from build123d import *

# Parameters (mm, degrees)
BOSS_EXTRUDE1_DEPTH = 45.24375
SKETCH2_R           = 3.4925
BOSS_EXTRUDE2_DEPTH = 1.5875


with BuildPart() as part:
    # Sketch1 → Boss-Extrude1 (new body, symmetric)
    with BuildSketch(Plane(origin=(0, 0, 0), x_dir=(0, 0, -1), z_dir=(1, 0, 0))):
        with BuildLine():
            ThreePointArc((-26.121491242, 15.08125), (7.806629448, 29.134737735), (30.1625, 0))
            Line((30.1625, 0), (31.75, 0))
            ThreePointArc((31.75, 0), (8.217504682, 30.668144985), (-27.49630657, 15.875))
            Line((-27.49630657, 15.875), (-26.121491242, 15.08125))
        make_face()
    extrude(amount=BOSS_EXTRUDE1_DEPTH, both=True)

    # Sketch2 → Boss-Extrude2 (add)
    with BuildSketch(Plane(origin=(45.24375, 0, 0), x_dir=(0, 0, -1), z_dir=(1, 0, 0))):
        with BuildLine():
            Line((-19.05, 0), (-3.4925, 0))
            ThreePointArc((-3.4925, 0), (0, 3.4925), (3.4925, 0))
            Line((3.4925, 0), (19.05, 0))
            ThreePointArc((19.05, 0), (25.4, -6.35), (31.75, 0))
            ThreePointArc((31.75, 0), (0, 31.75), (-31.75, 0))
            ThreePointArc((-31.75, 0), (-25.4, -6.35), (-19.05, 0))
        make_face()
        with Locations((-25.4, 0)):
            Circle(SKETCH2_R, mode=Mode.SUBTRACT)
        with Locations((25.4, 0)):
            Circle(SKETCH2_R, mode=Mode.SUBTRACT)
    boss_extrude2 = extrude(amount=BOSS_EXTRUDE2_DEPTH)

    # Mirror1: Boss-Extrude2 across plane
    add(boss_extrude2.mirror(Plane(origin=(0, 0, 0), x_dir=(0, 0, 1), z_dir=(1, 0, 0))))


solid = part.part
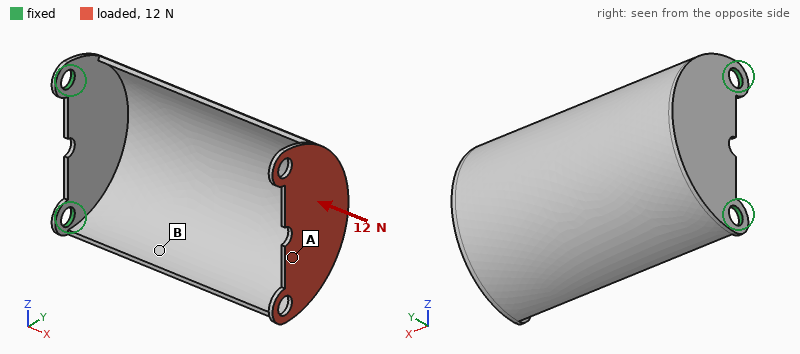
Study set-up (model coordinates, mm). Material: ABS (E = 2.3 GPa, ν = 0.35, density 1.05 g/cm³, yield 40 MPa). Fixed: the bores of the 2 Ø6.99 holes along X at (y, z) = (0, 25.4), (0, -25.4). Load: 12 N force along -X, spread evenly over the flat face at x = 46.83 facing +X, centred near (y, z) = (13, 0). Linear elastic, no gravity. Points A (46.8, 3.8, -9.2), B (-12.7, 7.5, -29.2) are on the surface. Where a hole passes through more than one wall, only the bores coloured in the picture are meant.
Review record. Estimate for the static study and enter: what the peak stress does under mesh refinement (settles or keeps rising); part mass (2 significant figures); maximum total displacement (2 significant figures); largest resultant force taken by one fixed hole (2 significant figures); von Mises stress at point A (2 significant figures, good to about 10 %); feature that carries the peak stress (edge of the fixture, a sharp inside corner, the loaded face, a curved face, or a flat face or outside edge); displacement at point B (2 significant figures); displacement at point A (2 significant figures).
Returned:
keeps rising
18 g
1.2 mm
6.1 N
1.3 MPa
edge of the fixture
0.24 mm
0.86 mm
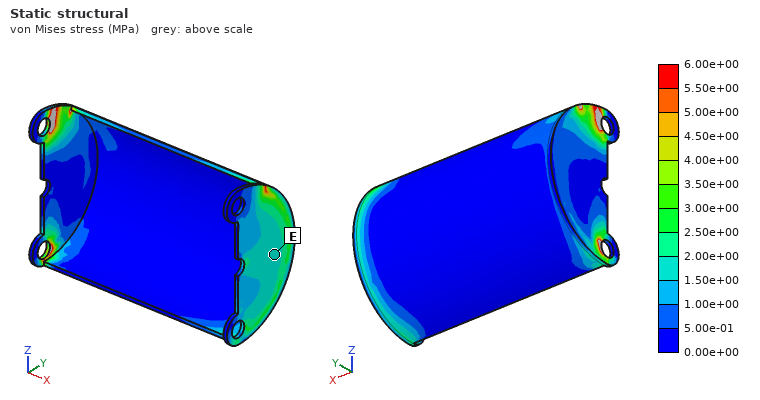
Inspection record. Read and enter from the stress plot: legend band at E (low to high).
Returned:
1.50e+00 to 2.00e+00 MPa
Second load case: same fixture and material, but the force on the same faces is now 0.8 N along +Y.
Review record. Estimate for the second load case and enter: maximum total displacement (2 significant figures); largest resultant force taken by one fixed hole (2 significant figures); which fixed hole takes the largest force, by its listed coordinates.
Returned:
1.3 mm
1.2 N
(0, 25.4)
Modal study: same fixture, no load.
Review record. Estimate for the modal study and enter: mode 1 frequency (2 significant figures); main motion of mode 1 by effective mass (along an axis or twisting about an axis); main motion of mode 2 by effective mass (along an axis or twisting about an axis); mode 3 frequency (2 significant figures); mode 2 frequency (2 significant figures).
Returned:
55 Hz
along Y
along Z
250 Hz
80 Hz
